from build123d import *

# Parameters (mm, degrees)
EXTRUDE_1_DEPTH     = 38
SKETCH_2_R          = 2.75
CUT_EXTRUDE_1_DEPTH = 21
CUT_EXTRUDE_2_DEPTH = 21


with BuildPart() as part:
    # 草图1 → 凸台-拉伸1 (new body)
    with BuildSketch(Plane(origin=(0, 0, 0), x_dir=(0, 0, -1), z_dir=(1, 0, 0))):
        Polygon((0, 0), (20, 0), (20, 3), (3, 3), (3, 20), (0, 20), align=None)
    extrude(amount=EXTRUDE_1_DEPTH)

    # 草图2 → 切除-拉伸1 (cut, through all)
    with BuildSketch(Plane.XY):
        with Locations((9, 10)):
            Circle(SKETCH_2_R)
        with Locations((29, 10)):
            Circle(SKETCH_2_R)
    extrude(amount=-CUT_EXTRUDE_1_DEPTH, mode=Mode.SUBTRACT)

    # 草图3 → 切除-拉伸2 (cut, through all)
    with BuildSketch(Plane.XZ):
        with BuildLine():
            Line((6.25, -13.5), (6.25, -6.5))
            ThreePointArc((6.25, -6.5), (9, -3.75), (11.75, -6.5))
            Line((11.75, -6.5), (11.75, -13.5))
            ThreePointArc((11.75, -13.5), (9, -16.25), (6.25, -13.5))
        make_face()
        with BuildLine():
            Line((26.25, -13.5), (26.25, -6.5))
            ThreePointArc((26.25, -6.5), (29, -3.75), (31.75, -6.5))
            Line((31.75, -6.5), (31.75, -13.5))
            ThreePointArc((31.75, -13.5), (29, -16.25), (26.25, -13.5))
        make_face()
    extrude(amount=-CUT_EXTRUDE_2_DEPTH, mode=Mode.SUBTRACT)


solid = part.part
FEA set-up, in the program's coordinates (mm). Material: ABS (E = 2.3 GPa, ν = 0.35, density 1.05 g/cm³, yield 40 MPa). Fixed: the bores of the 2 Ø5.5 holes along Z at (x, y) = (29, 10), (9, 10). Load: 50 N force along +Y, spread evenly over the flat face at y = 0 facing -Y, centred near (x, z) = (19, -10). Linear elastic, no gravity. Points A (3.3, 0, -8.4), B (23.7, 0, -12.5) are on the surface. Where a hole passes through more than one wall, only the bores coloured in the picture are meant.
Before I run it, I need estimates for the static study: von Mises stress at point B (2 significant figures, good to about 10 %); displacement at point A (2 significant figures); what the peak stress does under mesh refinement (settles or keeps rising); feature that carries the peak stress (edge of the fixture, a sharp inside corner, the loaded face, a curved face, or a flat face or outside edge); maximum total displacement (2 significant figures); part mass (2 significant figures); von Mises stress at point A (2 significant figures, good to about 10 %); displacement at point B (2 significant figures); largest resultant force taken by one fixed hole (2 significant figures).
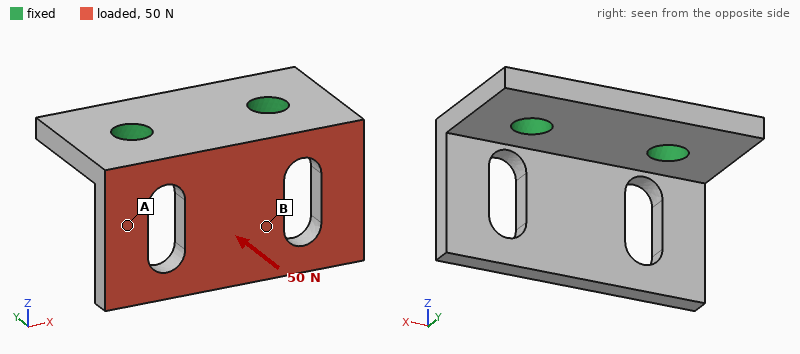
2.0 MPa
0.16 mm
keeps rising
edge of the fixture
0.48 mm
3.9 g
4.3 MPa
0.26 mm
25 N
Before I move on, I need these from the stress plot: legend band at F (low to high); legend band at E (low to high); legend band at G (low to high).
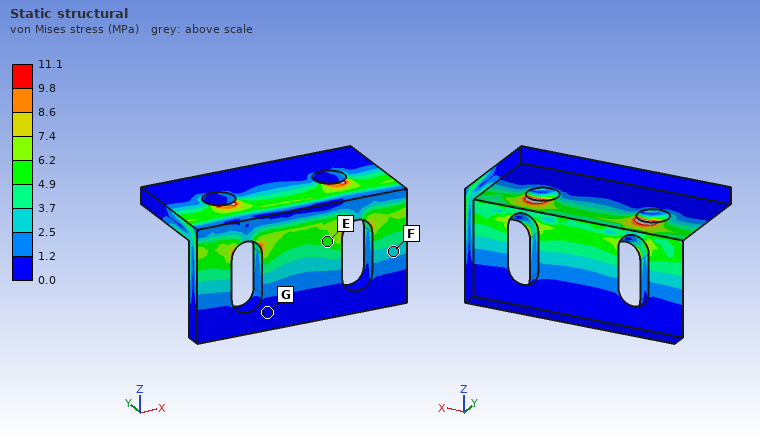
2.5 to 3.7 MPa
4.9 to 6.2 MPa
0.0 to 1.2 MPa
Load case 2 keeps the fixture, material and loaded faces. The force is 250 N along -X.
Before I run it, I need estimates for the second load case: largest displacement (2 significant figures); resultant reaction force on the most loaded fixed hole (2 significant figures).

0.29 mm
180 N
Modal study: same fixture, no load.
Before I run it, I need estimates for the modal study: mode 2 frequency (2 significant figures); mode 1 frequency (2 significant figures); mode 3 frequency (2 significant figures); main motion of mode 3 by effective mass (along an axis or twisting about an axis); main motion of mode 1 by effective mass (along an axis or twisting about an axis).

2200 Hz
1400 Hz
3700 Hz
along X
along Y
